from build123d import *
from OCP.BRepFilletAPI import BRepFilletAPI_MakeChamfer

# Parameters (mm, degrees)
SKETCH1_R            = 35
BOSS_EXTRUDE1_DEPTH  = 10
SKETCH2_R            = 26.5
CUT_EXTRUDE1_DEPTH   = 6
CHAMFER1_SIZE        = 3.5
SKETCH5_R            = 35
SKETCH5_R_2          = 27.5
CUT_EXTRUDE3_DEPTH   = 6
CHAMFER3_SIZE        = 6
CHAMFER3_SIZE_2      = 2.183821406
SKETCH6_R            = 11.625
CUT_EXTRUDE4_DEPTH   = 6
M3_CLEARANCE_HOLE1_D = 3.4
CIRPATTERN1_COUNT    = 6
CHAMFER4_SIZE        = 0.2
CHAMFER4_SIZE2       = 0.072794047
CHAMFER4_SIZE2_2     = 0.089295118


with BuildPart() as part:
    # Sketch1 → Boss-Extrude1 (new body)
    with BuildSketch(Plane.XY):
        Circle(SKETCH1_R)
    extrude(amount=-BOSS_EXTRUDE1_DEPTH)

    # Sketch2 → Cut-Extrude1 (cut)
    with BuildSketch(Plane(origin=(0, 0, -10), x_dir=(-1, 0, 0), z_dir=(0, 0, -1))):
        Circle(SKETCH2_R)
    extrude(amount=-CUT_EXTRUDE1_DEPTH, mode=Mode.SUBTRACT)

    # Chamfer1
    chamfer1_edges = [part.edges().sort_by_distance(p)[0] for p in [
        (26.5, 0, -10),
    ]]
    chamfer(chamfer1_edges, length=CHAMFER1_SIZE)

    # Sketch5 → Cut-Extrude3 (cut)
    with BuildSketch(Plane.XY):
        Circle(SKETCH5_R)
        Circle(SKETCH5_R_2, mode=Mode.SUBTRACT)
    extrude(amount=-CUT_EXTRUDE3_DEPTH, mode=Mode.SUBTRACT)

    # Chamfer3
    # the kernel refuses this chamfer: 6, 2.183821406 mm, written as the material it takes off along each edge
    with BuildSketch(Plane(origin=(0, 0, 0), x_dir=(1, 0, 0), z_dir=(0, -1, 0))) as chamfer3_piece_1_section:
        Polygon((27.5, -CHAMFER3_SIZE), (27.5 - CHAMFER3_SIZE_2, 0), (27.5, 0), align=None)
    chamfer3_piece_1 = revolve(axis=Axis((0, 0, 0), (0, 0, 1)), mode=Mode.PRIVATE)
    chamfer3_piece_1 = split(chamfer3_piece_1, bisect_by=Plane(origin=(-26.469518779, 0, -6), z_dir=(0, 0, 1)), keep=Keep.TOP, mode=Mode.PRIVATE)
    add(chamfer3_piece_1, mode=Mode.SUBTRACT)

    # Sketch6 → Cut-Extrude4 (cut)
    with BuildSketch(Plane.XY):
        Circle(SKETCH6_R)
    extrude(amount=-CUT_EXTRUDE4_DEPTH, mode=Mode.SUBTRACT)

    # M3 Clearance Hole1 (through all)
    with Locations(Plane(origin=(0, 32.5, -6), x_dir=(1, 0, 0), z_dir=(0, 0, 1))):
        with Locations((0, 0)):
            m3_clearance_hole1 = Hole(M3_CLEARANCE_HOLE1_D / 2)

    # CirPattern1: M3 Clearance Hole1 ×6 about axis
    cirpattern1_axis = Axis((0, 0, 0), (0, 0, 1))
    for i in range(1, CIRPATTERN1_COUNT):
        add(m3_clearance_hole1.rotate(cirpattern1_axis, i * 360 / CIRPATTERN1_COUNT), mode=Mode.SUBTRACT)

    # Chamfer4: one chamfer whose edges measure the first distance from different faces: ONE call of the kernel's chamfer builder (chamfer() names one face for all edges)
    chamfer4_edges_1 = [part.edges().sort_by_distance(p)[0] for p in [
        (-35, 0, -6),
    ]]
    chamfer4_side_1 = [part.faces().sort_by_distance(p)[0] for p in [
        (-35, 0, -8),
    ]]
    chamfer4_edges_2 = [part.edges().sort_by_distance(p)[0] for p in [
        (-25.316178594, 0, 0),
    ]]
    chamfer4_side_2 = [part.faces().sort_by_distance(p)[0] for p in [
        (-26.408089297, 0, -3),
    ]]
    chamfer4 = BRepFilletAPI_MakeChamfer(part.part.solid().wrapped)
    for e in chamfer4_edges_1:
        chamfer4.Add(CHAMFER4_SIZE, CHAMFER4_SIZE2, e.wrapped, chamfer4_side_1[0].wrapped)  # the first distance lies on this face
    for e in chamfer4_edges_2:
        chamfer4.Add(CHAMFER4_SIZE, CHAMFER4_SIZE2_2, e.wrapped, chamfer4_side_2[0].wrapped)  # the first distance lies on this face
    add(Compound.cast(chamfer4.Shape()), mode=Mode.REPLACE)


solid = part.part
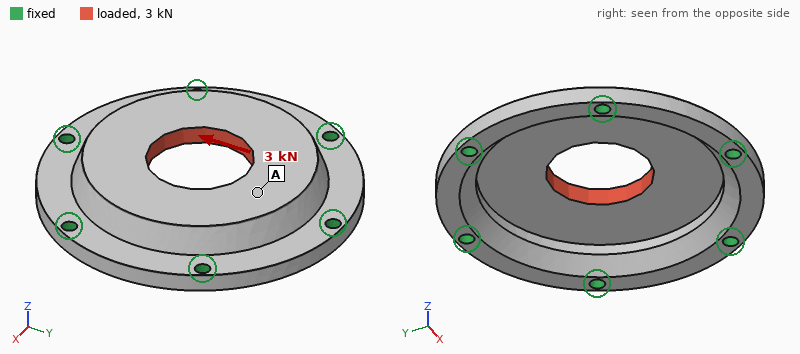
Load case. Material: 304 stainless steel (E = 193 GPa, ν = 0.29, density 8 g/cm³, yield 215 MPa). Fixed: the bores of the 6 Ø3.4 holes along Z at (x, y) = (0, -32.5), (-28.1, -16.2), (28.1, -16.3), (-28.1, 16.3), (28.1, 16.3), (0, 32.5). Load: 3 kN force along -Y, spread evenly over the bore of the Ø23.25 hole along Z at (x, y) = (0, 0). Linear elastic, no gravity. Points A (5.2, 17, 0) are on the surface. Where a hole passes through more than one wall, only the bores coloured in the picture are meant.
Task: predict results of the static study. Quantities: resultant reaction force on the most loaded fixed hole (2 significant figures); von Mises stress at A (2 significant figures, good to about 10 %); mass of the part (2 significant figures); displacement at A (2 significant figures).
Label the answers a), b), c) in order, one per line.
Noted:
a) 580 N
b) 16 MPa
c) 99 g
d) 5.4 µm
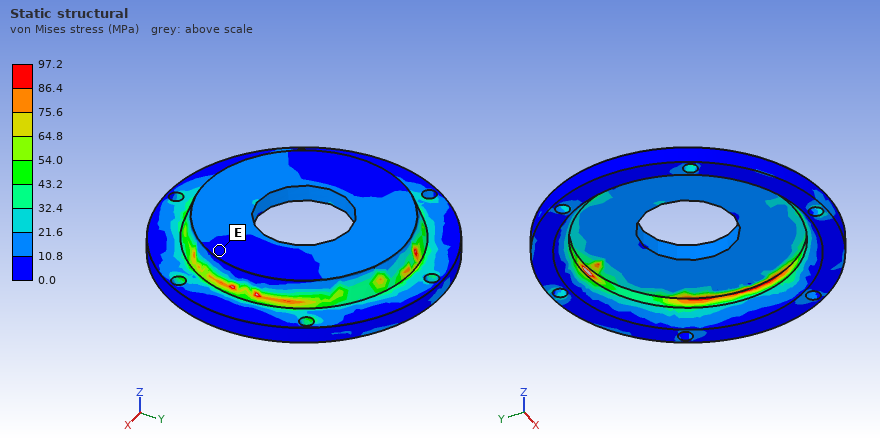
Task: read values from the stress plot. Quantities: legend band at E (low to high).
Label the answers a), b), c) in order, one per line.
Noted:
a) 0.0 to 10.8 MPa
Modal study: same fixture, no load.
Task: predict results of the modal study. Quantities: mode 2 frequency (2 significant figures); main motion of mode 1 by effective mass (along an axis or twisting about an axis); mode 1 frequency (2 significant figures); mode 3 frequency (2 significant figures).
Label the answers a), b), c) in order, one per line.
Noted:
a) 14 kHz
b) along Z
c) 8100 Hz
d) 14 kHz
